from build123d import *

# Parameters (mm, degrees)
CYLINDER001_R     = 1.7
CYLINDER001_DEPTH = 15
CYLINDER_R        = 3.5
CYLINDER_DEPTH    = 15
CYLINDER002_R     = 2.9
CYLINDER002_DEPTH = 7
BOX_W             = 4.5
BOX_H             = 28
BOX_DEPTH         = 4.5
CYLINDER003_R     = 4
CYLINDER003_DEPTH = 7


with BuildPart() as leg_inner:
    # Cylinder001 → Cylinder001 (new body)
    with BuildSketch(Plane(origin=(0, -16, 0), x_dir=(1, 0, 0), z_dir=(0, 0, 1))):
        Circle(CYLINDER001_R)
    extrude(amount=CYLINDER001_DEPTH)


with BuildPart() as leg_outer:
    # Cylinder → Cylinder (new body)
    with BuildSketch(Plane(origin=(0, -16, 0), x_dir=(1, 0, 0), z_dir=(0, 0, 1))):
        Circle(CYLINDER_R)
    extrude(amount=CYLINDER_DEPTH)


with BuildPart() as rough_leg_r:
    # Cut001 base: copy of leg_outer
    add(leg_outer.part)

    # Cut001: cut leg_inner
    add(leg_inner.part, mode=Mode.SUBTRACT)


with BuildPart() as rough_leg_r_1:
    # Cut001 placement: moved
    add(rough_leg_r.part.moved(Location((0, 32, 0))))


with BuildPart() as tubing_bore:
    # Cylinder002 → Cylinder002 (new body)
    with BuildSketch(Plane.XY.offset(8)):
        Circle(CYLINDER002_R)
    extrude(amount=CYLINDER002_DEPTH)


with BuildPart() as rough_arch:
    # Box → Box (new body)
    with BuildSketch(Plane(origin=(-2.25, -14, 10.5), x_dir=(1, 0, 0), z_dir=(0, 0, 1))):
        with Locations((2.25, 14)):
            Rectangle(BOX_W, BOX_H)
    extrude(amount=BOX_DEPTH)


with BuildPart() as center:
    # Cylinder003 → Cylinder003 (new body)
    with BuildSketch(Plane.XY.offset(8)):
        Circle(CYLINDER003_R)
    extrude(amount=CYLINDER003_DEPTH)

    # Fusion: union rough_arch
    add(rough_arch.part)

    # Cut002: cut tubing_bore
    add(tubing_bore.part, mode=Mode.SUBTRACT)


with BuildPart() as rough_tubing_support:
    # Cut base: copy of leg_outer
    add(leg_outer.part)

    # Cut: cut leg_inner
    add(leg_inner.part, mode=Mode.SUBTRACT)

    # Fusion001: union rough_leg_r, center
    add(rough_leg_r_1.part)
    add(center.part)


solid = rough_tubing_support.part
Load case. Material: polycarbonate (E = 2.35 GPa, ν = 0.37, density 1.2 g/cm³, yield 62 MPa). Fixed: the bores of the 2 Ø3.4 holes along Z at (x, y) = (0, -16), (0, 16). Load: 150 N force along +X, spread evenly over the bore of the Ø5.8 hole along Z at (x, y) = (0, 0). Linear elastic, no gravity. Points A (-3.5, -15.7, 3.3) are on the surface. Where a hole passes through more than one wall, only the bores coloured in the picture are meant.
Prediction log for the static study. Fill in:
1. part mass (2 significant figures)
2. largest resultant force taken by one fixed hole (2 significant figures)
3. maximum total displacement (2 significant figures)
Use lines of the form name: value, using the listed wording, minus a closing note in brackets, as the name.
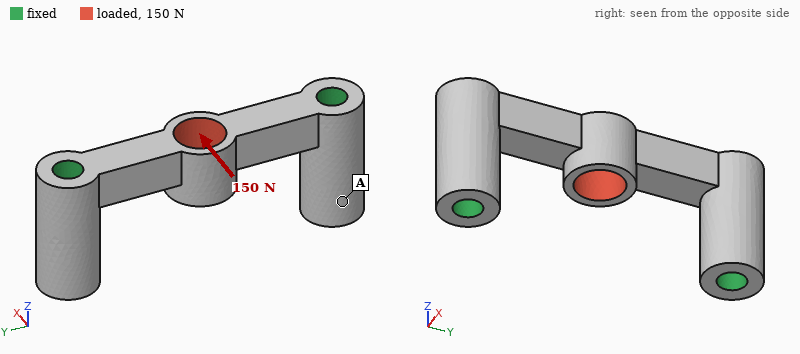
part mass: 1.7 g
largest resultant force taken by one fixed hole: 75 N
maximum total displacement: 0.38 mm
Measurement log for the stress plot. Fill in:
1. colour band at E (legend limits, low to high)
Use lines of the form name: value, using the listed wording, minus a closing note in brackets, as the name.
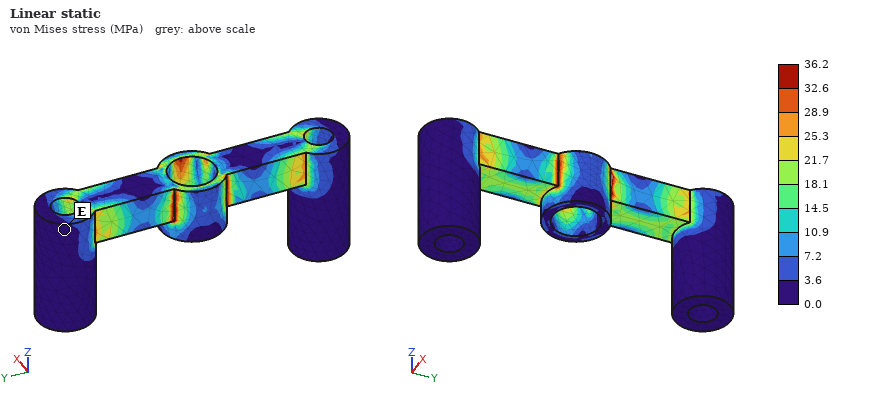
colour band at E: 0.0 to 3.6 MPa
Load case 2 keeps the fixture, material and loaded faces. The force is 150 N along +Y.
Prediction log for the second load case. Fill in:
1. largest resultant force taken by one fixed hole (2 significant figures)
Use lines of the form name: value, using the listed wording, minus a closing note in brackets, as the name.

largest resultant force taken by one fixed hole: 76 N
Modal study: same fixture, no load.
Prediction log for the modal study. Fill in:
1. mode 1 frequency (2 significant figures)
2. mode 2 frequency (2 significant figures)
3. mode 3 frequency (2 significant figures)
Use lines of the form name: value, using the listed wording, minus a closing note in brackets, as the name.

mode 1 frequency: 6100 Hz
mode 2 frequency: 6300 Hz
mode 3 frequency: 9400 Hz
